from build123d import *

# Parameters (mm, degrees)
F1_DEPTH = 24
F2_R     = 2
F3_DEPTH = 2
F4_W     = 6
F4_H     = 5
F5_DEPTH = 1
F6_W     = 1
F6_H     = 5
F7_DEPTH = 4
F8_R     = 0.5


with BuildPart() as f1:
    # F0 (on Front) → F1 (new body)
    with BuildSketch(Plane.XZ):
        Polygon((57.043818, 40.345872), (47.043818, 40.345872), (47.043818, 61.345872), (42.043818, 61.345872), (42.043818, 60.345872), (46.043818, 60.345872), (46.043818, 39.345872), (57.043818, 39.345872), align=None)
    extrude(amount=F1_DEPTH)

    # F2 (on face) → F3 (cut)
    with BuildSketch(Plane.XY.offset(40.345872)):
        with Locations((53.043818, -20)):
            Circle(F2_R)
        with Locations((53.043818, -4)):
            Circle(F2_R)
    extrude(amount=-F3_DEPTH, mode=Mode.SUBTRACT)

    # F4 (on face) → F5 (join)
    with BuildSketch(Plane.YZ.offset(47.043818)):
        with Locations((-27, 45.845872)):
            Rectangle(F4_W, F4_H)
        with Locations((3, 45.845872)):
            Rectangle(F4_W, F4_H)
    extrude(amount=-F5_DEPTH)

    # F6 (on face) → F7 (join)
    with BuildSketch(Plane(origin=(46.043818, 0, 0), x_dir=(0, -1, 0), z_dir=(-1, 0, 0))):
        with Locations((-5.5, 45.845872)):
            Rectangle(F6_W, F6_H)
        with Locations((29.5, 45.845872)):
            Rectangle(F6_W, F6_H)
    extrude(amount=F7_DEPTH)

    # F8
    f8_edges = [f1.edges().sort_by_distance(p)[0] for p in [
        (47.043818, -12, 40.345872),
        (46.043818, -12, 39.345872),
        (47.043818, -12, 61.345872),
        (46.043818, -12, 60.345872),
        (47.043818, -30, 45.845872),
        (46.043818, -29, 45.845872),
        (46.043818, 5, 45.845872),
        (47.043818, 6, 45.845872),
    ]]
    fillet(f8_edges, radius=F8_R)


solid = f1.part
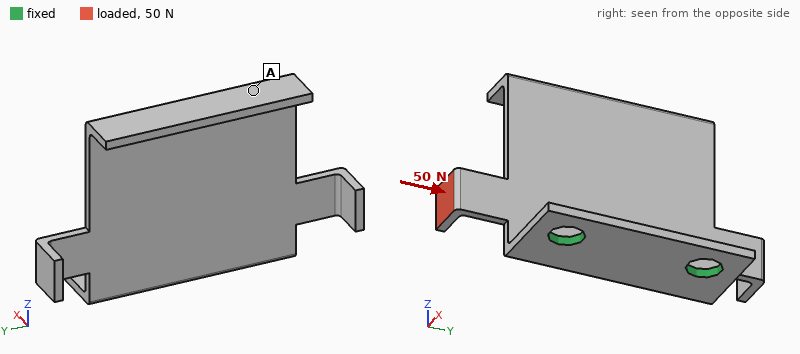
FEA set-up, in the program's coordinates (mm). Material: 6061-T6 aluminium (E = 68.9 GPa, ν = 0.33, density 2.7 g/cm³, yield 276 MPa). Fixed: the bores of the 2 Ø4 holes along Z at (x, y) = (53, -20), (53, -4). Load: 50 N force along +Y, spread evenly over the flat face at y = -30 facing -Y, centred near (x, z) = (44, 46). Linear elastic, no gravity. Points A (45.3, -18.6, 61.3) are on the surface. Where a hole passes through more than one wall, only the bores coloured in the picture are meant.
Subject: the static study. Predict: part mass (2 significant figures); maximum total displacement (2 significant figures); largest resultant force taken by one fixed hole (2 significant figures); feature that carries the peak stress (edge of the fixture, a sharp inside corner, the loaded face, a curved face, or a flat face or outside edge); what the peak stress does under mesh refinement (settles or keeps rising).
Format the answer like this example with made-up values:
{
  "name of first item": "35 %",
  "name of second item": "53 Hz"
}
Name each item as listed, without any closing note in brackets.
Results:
{
  "part mass": "2.5 g",
  "maximum total displacement": "0.21 mm",
  "largest resultant force taken by one fixed hole": "38 N",
  "feature that carries the peak stress": "a sharp inside corner",
  "what the peak stress does under mesh refinement": "keeps rising"
}
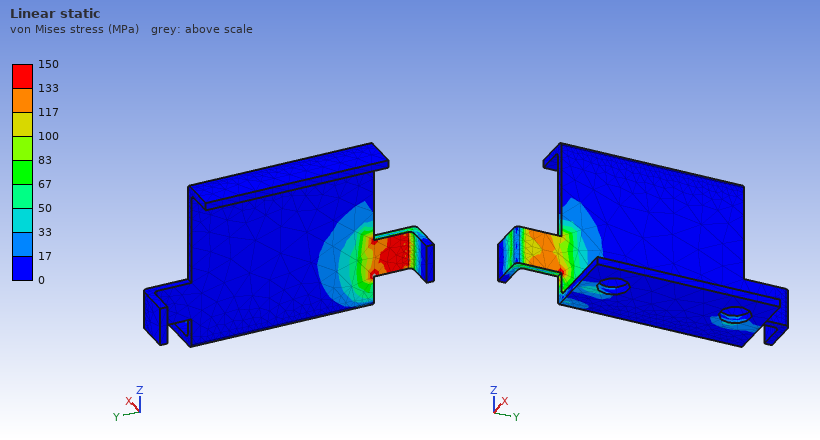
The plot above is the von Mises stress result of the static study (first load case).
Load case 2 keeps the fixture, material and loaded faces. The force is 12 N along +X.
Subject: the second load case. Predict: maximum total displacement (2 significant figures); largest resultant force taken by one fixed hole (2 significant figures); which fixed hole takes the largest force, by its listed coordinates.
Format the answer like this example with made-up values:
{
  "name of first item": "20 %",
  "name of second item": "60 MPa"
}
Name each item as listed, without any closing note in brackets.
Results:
{
  "maximum total displacement": "0.19 mm",
  "largest resultant force taken by one fixed hole": "18 N",
  "which fixed hole takes the largest force, by its listed coordinates": "(53, -20)"
}
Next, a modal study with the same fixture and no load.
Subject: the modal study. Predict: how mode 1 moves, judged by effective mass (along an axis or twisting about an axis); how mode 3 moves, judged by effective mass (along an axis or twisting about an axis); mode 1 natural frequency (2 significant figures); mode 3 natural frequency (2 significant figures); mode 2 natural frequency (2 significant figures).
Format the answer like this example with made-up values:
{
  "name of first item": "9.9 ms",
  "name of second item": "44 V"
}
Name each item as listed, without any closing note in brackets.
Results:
{
  "how mode 1 moves, judged by effective mass": "along X",
  "how mode 3 moves, judged by effective mass": "along Y",
  "mode 1 natural frequency": "1000 Hz",
  "mode 3 natural frequency": "4200 Hz",
  "mode 2 natural frequency": "2700 Hz"
}
